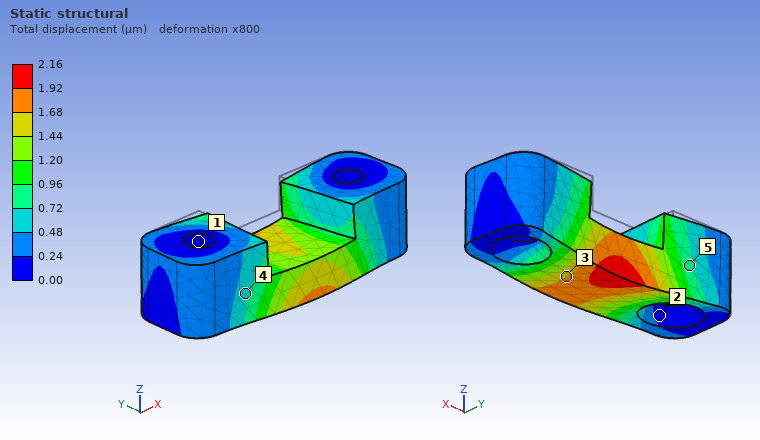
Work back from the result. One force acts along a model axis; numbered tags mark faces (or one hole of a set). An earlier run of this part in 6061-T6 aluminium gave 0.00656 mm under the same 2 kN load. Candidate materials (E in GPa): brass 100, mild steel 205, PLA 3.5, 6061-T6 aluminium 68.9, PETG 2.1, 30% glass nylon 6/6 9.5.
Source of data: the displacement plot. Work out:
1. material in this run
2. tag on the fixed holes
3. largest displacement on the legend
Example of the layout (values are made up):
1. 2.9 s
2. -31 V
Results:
1. mild steel
2. 1
3. 2.16 µm
